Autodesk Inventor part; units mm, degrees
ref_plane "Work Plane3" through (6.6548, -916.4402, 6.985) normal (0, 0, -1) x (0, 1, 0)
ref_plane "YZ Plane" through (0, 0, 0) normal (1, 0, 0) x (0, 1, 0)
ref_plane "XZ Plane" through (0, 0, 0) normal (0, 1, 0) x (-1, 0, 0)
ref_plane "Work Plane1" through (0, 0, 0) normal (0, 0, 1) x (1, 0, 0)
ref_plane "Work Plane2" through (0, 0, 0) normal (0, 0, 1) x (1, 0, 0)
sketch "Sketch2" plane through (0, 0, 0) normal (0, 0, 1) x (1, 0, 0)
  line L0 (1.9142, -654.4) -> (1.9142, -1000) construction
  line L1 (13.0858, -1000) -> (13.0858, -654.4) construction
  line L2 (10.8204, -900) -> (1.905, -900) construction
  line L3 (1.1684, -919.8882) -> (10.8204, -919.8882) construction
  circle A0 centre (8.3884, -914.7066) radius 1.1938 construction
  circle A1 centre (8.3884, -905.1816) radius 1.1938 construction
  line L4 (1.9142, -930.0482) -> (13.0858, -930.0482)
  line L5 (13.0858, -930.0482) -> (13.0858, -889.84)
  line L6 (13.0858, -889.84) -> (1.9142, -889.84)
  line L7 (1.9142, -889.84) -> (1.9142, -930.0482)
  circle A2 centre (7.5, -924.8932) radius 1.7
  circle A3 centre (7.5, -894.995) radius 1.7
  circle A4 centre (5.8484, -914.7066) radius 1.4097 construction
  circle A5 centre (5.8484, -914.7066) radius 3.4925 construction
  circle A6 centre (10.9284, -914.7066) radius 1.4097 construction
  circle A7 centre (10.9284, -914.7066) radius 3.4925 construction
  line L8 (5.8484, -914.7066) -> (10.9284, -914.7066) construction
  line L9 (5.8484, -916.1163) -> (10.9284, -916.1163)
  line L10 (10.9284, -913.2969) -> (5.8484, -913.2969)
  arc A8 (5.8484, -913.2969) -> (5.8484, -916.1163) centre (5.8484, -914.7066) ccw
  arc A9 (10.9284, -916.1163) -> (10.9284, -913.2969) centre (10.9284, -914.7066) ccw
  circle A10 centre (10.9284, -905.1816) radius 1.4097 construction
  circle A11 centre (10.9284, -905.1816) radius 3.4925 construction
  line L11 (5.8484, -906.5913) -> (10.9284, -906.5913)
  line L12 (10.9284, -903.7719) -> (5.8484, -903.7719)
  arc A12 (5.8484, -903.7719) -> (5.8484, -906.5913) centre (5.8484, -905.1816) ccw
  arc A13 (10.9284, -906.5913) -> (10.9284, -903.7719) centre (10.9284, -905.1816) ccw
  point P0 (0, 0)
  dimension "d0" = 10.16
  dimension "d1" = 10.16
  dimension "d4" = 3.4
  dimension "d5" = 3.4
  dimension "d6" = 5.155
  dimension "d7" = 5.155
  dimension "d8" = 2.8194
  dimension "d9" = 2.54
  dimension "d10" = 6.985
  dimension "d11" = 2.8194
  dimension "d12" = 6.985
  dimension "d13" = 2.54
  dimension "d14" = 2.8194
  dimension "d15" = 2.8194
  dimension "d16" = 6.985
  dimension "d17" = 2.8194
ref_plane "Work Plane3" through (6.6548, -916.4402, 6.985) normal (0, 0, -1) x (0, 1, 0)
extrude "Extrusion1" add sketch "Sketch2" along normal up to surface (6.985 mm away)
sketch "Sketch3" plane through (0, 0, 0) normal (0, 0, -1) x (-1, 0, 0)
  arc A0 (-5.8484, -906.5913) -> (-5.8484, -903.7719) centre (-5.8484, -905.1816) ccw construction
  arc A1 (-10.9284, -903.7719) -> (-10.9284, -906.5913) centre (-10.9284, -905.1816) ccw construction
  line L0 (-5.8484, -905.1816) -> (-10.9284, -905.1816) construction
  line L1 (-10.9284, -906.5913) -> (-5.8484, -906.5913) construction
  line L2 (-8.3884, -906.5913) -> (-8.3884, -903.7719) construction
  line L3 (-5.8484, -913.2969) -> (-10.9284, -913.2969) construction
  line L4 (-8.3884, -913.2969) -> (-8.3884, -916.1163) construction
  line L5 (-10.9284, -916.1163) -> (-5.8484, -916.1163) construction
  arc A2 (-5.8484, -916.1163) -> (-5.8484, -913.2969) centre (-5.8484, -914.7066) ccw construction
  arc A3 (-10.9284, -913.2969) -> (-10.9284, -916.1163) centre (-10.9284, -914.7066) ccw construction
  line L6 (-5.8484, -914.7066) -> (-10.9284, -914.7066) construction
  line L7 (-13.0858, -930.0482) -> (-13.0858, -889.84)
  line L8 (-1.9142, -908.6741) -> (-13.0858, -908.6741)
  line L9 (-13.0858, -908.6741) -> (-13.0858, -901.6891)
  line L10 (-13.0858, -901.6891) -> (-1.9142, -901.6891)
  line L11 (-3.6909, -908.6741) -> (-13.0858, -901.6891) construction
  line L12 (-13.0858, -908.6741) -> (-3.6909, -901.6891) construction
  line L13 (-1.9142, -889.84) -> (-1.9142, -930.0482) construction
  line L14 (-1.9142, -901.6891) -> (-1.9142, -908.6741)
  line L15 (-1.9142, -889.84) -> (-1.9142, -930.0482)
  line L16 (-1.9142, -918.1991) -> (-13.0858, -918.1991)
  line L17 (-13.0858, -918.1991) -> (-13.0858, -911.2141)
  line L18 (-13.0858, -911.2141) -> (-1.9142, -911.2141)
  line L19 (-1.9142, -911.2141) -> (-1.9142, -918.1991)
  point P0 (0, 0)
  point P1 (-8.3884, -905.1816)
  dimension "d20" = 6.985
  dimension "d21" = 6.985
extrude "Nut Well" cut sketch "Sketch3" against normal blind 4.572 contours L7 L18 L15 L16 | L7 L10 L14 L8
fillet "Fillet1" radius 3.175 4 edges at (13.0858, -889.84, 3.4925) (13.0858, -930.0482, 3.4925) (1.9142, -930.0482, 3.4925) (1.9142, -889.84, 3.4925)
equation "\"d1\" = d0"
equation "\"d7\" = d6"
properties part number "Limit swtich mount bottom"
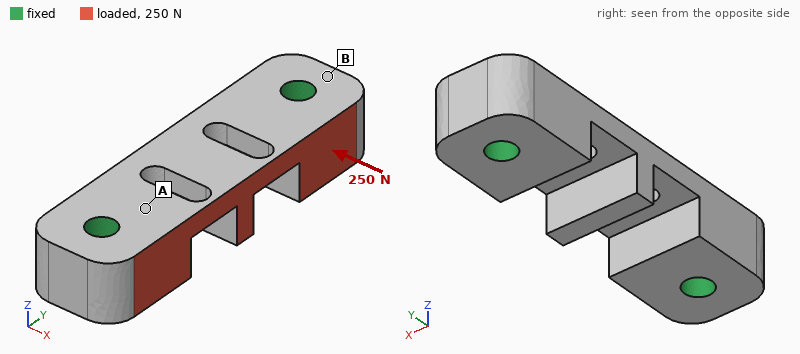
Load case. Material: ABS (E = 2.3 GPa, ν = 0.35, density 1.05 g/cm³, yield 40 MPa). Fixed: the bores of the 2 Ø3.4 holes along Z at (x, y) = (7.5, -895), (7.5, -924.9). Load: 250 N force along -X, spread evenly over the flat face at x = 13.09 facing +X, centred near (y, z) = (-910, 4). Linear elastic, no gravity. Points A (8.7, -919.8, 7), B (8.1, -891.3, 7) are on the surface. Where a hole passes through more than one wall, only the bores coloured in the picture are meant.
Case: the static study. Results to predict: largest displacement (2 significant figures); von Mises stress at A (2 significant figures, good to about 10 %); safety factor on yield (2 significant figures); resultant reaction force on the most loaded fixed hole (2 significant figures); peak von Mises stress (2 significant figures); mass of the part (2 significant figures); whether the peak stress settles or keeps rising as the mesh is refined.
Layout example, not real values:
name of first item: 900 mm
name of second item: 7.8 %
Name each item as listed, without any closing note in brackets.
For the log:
largest displacement: 0.11 mm
von Mises stress at A: 3.1 MPa
safety factor on yield: 1.7
resultant reaction force on the most loaded fixed hole: 130 N
peak von Mises stress: 23 MPa
mass of the part: 2.2 g
whether the peak stress settles or keeps rising as the mesh is refined: settles
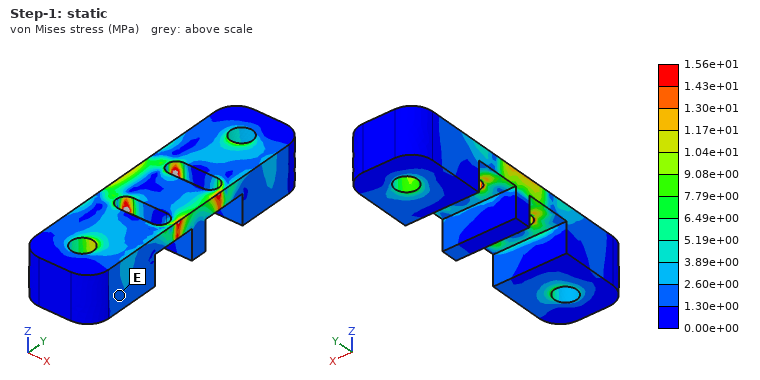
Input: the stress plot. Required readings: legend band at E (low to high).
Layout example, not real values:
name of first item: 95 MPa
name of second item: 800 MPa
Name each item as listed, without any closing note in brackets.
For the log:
legend band at E: 1.30e+00 to 2.60e+00 MPa
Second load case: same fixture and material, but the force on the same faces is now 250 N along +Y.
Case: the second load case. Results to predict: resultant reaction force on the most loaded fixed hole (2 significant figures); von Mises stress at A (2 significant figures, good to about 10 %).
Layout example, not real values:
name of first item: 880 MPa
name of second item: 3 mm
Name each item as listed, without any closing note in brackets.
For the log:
resultant reaction force on the most loaded fixed hole: 130 N
von Mises stress at A: 3.0 MPa
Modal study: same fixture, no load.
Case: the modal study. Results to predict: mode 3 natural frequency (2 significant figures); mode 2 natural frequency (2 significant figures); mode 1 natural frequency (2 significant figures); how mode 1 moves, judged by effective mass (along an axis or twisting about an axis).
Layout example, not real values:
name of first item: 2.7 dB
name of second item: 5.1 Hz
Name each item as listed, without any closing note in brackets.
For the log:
mode 3 natural frequency: 8900 Hz
mode 2 natural frequency: 6500 Hz
mode 1 natural frequency: 5700 Hz
how mode 1 moves, judged by effective mass: along Z
